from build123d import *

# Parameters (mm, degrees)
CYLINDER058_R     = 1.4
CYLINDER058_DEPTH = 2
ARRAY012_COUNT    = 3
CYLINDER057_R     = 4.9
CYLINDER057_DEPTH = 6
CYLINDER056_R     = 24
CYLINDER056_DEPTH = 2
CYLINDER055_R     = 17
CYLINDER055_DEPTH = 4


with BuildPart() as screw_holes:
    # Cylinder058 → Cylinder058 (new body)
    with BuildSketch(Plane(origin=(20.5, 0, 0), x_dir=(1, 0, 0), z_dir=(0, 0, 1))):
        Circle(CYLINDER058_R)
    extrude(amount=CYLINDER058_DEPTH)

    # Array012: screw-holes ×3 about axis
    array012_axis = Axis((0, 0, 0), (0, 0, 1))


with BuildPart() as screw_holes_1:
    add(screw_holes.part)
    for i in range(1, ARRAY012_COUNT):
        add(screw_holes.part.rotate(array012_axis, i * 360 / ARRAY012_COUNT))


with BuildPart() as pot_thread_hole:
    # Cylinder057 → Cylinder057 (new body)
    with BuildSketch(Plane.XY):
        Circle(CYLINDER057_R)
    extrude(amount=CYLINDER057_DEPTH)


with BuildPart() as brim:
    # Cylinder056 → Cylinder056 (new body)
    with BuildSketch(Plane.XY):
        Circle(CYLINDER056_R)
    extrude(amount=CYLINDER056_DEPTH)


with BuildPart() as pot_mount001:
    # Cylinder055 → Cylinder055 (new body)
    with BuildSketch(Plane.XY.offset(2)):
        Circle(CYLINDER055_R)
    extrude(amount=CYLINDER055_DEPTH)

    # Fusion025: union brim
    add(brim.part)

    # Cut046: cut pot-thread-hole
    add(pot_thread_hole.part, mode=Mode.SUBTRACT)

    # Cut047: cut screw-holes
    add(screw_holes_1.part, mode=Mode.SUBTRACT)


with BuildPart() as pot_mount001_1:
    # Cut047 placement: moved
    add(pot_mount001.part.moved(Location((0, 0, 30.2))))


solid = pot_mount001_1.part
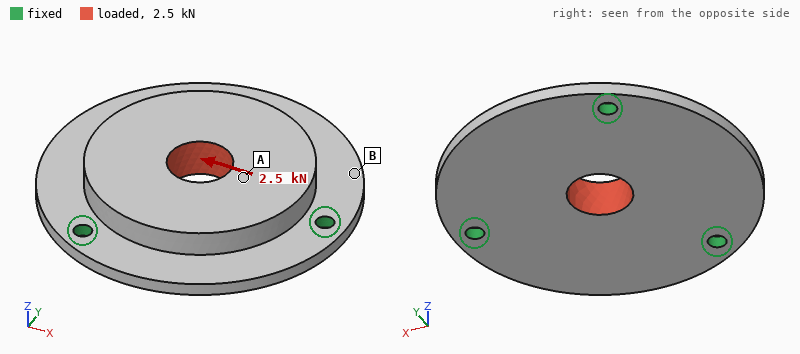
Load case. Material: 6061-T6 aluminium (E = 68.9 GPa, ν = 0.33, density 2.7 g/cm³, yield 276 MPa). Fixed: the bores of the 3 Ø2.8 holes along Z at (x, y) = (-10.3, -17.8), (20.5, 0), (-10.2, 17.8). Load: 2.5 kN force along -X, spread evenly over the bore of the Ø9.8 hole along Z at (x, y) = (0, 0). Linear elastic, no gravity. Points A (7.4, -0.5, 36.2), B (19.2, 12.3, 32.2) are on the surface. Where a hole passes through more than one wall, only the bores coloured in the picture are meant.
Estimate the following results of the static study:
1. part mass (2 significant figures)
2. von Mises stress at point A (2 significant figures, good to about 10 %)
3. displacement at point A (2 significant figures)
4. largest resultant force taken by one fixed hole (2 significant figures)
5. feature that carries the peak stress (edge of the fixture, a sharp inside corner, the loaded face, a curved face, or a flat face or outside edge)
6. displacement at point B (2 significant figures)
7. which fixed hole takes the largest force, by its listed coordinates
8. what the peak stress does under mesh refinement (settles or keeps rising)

18 g
20 MPa
6.7 µm
980 N
edge of the fixture
5.9 µm
(20.5, 0)
keeps rising
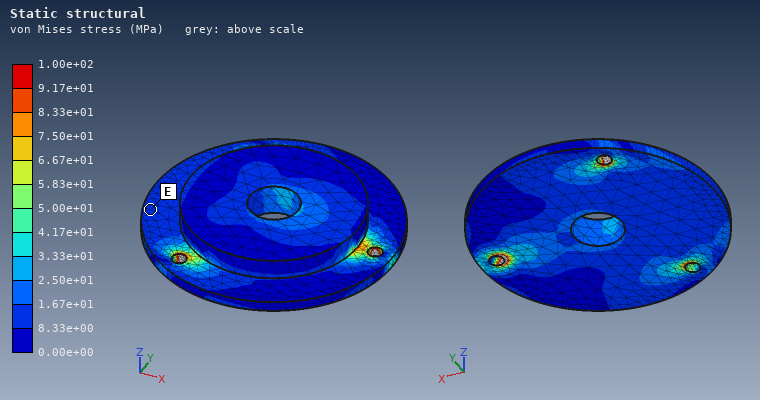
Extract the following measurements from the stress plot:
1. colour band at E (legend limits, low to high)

8.33e+00 to 1.67e+01 MPa
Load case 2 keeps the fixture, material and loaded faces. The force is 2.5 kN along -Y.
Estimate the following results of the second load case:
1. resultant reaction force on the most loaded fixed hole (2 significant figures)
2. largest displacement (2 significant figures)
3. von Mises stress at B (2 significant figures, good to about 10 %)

920 N
9.7 µm
12 MPa
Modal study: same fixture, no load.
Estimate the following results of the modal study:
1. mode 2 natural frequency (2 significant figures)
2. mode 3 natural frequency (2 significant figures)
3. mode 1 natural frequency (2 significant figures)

10 kHz
11 kHz
10 kHz
